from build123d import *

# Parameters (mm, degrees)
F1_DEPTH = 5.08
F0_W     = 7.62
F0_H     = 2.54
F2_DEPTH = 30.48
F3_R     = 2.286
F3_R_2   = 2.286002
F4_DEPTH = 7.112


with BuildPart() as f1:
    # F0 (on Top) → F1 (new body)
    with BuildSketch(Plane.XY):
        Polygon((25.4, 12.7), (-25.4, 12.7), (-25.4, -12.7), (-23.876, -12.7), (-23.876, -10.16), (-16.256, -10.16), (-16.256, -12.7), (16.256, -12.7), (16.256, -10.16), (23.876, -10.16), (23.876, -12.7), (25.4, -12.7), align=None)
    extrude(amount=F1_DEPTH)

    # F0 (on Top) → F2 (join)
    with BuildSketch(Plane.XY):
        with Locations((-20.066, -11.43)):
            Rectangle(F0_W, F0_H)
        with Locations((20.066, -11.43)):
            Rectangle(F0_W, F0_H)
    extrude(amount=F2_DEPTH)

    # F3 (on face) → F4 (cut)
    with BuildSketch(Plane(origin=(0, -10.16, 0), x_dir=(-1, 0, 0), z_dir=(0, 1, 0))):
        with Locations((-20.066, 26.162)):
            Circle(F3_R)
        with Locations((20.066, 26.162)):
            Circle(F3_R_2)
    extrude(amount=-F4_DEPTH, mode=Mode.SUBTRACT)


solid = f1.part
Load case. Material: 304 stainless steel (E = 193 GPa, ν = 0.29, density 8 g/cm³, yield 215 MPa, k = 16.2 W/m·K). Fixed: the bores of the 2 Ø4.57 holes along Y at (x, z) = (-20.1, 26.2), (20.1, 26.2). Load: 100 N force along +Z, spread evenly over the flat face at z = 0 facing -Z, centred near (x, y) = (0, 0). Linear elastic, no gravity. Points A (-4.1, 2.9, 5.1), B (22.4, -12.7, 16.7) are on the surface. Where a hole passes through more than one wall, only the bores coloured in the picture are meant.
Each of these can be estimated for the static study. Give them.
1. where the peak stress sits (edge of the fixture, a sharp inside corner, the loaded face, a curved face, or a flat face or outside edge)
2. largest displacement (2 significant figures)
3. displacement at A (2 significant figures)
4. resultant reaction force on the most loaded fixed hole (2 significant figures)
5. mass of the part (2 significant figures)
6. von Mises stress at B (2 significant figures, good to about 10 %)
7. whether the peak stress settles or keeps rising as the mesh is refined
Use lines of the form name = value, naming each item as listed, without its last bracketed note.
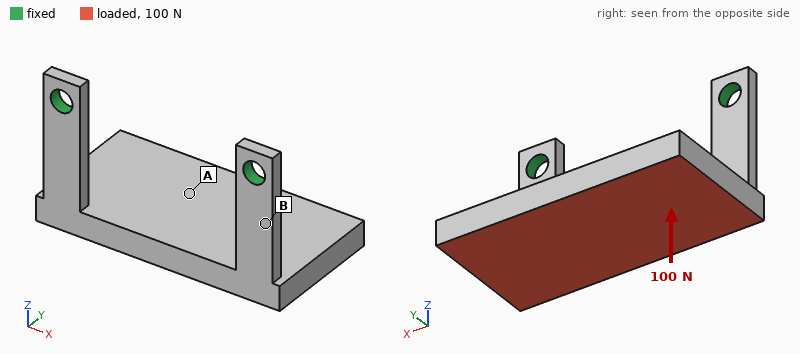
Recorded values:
where the peak stress sits = edge of the fixture
largest displacement = 0.16 mm
displacement at A = 0.099 mm
resultant reaction force on the most loaded fixed hole = 51 N
mass of the part = 60 g
von Mises stress at B = 67 MPa
whether the peak stress settles or keeps rising as the mesh is refined = keeps rising
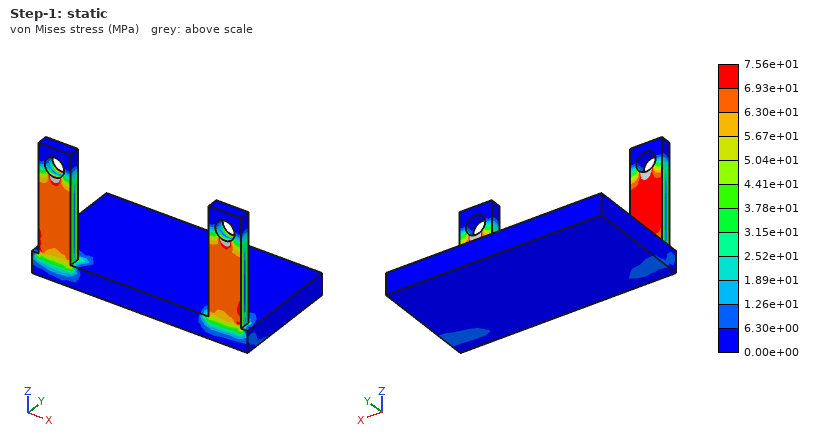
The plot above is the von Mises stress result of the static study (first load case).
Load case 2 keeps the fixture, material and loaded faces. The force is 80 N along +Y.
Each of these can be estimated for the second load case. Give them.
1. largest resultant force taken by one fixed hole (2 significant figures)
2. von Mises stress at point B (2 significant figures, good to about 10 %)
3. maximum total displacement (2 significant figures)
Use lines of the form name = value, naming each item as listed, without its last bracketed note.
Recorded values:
largest resultant force taken by one fixed hole = 40 N
von Mises stress at point B = 81 MPa
maximum total displacement = 0.17 mm
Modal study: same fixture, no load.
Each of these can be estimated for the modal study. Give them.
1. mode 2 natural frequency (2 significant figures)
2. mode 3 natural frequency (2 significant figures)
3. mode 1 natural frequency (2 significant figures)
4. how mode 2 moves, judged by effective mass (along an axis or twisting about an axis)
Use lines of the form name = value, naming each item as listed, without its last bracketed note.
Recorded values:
mode 2 natural frequency = 1500 Hz
mode 3 natural frequency = 2100 Hz
mode 1 natural frequency = 530 Hz
how mode 2 moves, judged by effective mass = along X
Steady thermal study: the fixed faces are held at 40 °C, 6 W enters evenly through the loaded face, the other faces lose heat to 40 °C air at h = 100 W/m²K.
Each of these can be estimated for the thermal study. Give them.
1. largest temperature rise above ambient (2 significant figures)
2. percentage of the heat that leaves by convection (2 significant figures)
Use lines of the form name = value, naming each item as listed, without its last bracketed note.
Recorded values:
largest temperature rise above ambient = 27 K
percentage of the heat that leaves by convection = 93 %
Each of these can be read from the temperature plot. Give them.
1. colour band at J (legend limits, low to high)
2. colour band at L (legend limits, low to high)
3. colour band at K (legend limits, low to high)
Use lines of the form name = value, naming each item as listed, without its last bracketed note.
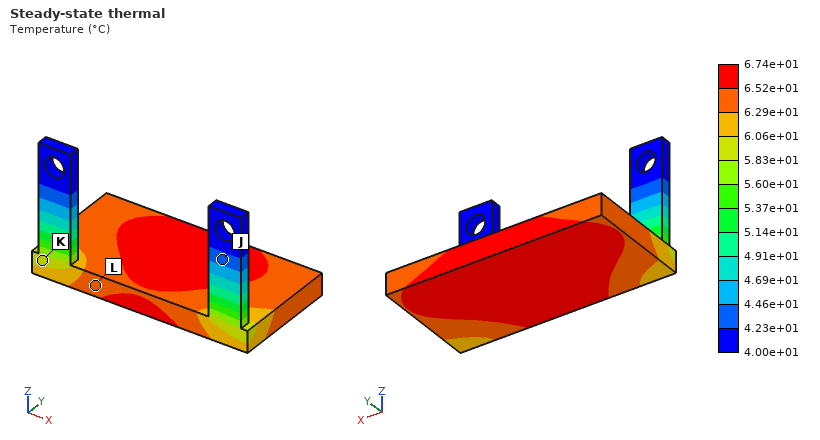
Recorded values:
colour band at J = 4.23e+01 to 4.46e+01 °C
colour band at L = 6.29e+01 to 6.52e+01 °C
colour band at K = 5.83e+01 to 6.06e+01 °C
